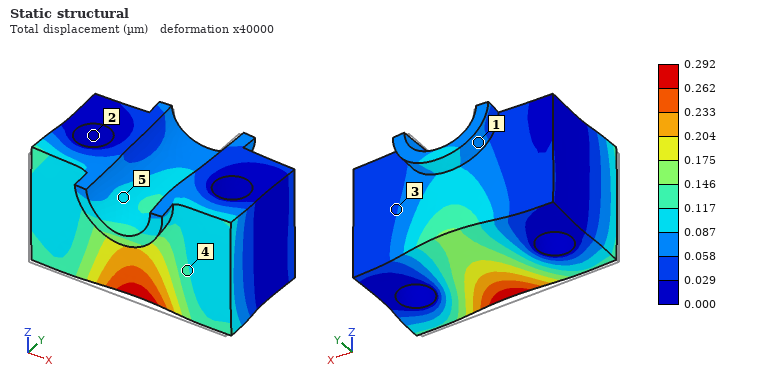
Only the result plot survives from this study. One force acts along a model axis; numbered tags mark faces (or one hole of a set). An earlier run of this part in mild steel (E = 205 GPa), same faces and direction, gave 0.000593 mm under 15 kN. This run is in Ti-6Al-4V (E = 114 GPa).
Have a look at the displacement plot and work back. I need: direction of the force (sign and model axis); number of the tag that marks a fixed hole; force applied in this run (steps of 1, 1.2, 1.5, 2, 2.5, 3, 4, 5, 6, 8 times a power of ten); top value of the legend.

+Y
2
4 kN
0.292 µm
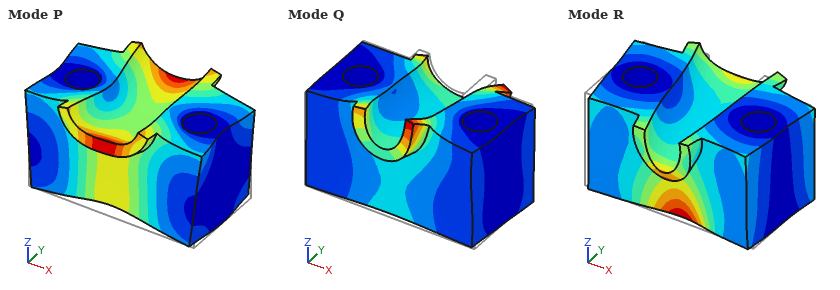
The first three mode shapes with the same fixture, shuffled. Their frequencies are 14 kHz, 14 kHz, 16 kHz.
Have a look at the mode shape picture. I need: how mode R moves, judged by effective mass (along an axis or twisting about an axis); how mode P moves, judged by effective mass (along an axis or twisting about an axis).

along Y
along Z
